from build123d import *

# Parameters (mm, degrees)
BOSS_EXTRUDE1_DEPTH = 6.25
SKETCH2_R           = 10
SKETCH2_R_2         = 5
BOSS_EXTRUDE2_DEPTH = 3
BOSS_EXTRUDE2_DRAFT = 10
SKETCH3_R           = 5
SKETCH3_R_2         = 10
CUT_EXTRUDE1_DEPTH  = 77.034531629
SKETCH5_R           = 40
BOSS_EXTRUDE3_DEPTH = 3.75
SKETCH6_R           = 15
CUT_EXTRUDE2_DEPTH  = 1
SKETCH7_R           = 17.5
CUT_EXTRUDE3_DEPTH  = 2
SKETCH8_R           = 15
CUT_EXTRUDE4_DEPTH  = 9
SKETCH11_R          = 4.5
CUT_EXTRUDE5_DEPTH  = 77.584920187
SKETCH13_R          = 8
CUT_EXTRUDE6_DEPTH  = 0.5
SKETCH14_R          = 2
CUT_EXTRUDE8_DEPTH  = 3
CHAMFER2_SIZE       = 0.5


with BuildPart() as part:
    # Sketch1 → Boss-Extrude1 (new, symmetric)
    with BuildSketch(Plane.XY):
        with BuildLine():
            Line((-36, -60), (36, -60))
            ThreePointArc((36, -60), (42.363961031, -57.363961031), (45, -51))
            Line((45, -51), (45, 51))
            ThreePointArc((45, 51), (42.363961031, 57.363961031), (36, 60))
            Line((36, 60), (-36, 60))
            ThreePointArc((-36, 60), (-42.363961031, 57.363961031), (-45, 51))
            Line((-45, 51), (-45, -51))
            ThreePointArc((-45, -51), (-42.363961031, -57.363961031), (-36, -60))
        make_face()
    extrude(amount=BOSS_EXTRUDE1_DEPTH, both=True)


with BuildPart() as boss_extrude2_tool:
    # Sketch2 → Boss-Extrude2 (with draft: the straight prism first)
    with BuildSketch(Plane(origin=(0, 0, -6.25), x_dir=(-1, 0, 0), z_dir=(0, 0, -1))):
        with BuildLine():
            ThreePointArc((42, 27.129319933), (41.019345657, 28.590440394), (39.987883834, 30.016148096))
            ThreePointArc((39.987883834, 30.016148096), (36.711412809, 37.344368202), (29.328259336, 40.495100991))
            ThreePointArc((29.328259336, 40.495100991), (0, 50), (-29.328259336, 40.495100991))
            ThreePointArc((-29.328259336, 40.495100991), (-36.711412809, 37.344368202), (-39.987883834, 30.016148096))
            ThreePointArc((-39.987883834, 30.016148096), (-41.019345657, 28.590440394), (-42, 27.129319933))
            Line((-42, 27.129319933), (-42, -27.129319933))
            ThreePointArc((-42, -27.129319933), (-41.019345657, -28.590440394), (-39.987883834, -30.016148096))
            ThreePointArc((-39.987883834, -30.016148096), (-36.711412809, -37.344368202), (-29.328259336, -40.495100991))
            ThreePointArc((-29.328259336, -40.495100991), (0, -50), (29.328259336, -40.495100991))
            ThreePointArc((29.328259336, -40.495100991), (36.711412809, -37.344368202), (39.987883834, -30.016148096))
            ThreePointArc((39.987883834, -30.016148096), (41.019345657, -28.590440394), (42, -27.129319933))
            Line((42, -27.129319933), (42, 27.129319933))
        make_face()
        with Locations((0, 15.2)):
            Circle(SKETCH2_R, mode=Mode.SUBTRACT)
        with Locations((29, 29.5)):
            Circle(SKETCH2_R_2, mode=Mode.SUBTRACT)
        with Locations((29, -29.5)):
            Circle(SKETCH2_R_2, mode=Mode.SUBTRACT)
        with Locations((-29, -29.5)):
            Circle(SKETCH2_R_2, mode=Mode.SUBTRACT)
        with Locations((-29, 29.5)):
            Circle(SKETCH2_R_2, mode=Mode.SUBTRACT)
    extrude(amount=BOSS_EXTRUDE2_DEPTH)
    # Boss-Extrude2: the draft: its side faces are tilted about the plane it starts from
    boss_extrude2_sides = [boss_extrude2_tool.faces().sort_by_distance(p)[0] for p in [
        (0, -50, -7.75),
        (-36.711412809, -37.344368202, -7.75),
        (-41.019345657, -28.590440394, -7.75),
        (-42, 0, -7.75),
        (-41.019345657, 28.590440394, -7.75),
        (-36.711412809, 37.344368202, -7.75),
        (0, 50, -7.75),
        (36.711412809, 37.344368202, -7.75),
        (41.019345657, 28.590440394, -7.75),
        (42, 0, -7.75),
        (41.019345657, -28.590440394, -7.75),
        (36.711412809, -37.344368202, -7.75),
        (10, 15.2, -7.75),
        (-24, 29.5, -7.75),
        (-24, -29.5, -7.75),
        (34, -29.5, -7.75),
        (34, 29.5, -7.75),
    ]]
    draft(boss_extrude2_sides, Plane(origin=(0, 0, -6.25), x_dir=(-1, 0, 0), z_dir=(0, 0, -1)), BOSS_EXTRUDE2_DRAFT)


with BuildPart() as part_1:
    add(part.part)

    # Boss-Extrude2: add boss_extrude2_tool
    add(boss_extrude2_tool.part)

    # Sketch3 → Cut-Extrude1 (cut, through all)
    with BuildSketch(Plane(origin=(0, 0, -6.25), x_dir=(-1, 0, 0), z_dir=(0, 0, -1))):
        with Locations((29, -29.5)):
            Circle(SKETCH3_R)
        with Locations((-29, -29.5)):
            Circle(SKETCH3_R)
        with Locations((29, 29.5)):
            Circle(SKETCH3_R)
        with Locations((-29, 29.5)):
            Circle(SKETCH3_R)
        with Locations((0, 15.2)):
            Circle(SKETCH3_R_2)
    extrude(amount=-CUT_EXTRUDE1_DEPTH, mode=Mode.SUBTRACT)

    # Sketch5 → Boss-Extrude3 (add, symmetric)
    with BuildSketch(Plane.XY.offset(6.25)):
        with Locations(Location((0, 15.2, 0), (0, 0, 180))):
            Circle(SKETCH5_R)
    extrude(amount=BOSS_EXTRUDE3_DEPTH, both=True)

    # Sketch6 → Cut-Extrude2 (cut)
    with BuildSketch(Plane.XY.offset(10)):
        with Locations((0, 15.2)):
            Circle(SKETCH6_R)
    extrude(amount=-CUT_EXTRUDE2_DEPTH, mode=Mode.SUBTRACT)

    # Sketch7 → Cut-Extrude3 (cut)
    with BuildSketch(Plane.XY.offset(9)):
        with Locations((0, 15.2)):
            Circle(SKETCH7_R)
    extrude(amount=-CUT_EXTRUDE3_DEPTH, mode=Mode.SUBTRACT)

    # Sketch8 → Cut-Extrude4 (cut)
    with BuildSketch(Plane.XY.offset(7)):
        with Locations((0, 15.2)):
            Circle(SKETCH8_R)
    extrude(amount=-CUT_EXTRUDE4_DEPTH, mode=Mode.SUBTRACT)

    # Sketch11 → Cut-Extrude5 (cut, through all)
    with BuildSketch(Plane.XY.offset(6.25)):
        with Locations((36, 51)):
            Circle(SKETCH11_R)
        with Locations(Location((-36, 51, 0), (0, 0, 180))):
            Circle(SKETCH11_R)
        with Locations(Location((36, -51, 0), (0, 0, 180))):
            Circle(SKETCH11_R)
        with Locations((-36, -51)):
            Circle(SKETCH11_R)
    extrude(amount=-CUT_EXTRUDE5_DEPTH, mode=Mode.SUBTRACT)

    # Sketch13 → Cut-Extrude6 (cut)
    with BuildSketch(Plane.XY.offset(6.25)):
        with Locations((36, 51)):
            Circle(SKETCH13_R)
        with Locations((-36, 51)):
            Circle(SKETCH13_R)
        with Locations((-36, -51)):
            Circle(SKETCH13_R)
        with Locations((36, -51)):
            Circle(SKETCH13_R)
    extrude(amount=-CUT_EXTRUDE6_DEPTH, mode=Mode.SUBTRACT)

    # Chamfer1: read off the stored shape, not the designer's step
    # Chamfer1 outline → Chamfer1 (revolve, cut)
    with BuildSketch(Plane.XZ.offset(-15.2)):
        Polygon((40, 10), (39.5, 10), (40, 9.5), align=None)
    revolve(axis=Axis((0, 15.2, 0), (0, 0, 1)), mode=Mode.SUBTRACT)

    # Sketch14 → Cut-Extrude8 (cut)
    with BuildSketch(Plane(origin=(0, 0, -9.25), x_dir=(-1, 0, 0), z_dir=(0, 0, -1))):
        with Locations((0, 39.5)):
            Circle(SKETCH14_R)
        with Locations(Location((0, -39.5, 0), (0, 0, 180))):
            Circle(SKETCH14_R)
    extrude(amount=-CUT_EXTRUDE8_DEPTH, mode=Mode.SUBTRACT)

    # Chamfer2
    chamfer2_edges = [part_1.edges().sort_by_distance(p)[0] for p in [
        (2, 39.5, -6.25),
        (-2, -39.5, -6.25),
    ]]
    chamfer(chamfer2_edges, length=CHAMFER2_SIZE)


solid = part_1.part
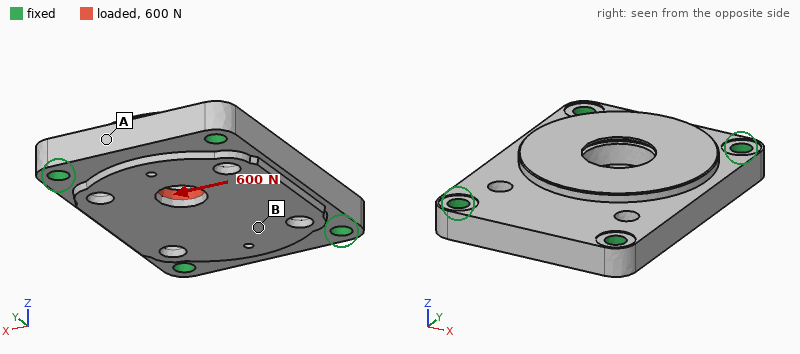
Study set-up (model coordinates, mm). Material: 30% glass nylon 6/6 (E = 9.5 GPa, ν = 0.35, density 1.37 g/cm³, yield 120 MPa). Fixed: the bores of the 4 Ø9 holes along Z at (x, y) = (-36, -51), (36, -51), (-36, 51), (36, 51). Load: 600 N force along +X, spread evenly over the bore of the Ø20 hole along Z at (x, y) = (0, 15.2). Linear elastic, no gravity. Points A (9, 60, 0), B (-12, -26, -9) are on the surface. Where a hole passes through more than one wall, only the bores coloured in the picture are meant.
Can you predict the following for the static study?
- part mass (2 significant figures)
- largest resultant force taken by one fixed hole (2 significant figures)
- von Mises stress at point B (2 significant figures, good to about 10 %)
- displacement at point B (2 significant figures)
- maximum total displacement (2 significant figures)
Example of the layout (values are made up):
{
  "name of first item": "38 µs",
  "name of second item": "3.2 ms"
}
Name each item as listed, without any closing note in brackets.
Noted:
{
  "part mass": "210 g",
  "largest resultant force taken by one fixed hole": "210 N",
  "von Mises stress at point B": "0.48 MPa",
  "displacement at point B": "2.1 µm",
  "maximum total displacement": "6.2 µm"
}
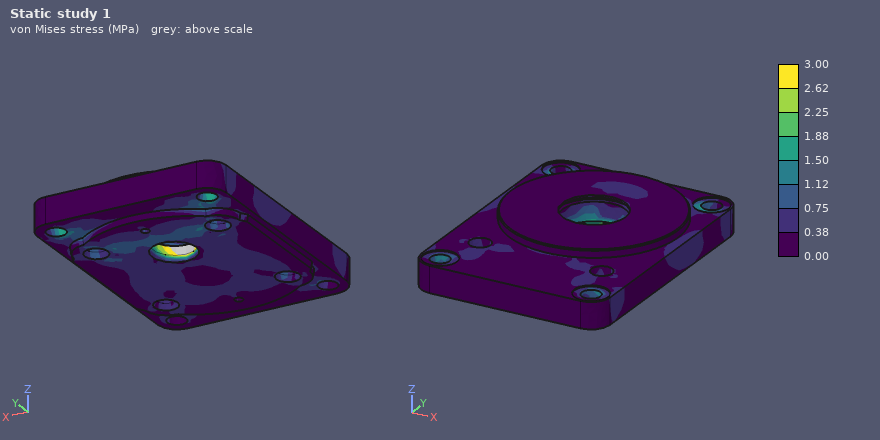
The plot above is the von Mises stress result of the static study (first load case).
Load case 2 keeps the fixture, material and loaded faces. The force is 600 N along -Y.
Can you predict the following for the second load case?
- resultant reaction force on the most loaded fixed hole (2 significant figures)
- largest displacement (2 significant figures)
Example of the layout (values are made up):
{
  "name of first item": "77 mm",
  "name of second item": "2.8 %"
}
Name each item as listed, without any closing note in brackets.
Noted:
{
  "resultant reaction force on the most loaded fixed hole": "190 N",
  "largest displacement": "4.9 µm"
}
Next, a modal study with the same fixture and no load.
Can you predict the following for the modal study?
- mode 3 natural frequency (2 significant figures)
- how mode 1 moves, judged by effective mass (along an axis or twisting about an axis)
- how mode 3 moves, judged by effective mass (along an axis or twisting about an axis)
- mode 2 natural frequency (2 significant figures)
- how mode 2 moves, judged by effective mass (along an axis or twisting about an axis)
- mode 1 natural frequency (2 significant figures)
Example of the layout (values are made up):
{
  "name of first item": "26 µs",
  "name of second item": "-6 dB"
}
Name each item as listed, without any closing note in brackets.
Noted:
{
  "mode 3 natural frequency": "5700 Hz",
  "how mode 1 moves, judged by effective mass": "along Z",
  "how mode 3 moves, judged by effective mass": "twisting about X",
  "mode 2 natural frequency": "3900 Hz",
  "how mode 2 moves, judged by effective mass": "twisting about Y",
  "mode 1 natural frequency": "2700 Hz"
}
